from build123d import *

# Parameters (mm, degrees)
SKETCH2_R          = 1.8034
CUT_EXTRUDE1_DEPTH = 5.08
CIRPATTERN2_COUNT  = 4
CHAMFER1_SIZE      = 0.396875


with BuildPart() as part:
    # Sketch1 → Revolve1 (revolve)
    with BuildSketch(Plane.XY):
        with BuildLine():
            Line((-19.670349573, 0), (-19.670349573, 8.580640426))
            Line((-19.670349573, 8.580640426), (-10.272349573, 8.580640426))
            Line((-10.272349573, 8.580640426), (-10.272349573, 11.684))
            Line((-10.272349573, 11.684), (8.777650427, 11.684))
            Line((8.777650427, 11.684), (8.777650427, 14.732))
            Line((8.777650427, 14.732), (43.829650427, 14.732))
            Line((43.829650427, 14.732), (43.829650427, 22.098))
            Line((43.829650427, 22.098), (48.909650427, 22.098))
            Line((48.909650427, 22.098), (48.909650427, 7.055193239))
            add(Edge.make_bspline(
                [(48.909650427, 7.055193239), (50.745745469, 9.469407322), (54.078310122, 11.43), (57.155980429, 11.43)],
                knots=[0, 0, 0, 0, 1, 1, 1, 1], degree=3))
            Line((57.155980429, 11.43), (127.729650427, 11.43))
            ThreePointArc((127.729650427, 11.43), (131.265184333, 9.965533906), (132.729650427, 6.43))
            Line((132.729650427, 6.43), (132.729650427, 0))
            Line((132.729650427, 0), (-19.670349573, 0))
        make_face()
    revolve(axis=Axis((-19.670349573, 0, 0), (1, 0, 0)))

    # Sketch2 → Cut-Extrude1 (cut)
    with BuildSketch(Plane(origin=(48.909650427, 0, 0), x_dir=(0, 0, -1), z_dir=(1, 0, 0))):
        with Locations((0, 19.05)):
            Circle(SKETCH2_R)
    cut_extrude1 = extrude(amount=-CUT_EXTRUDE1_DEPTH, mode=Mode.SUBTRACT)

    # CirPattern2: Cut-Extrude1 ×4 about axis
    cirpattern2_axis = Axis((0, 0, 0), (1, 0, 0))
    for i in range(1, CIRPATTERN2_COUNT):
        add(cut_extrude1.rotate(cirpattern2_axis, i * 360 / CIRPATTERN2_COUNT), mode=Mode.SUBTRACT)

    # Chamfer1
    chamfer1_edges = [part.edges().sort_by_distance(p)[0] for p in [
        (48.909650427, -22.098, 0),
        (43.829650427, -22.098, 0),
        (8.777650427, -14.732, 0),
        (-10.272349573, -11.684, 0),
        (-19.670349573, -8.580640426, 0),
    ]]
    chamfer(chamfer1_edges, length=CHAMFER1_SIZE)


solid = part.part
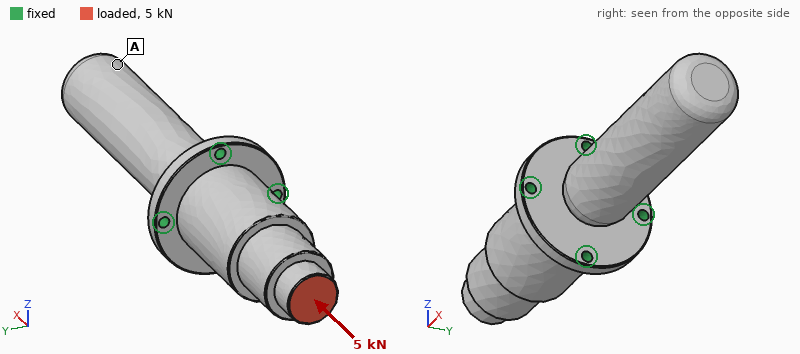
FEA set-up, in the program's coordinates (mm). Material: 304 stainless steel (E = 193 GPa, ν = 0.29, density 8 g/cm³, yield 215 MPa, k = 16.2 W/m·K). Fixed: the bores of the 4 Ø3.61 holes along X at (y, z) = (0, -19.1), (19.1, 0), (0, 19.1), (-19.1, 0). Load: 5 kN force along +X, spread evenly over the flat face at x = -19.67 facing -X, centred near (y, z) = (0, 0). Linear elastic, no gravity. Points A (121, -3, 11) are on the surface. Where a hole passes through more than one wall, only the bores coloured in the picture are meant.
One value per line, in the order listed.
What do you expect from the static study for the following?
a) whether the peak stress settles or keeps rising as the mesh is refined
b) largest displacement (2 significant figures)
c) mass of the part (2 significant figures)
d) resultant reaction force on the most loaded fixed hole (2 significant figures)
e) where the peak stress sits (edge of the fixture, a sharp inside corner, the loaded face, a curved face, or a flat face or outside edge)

keeps rising
6.7 µm
600 g
1.3 kN
edge of the fixture
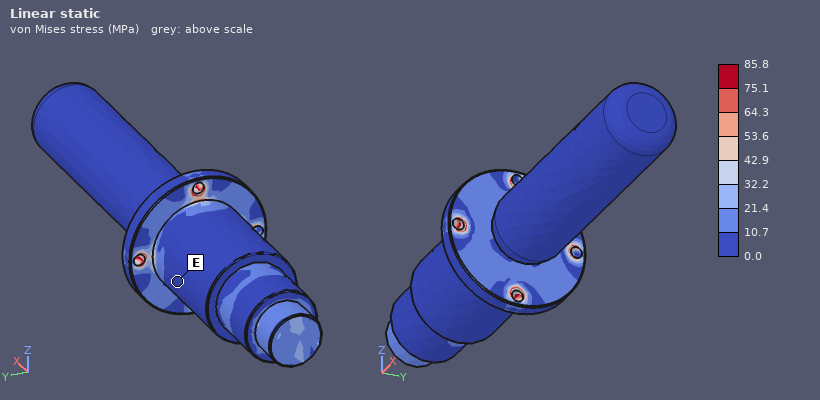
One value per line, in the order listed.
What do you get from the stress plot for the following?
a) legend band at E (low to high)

0.0 to 10.7 MPa
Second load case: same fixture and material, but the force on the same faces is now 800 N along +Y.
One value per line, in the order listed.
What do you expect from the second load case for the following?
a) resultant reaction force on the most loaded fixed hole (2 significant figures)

1.5 kN
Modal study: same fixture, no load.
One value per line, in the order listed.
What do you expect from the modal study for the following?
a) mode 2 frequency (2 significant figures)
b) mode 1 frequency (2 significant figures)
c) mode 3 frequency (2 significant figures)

1200 Hz
1200 Hz
3900 Hz
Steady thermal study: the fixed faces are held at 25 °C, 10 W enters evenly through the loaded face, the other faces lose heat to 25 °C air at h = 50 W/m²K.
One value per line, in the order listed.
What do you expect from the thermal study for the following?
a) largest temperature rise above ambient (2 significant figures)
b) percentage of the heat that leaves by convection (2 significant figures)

67 K
69 %
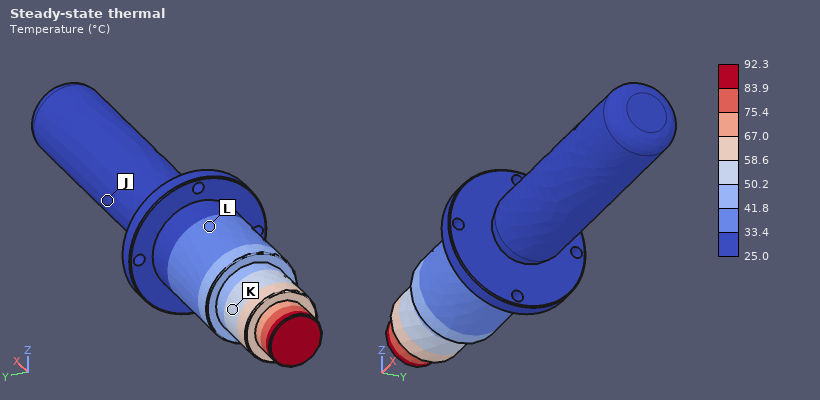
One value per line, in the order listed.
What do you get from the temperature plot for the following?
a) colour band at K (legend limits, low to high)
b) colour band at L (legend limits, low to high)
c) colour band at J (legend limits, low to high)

50.2 to 58.6 °C
33.4 to 41.8 °C
25.0 to 33.4 °C
